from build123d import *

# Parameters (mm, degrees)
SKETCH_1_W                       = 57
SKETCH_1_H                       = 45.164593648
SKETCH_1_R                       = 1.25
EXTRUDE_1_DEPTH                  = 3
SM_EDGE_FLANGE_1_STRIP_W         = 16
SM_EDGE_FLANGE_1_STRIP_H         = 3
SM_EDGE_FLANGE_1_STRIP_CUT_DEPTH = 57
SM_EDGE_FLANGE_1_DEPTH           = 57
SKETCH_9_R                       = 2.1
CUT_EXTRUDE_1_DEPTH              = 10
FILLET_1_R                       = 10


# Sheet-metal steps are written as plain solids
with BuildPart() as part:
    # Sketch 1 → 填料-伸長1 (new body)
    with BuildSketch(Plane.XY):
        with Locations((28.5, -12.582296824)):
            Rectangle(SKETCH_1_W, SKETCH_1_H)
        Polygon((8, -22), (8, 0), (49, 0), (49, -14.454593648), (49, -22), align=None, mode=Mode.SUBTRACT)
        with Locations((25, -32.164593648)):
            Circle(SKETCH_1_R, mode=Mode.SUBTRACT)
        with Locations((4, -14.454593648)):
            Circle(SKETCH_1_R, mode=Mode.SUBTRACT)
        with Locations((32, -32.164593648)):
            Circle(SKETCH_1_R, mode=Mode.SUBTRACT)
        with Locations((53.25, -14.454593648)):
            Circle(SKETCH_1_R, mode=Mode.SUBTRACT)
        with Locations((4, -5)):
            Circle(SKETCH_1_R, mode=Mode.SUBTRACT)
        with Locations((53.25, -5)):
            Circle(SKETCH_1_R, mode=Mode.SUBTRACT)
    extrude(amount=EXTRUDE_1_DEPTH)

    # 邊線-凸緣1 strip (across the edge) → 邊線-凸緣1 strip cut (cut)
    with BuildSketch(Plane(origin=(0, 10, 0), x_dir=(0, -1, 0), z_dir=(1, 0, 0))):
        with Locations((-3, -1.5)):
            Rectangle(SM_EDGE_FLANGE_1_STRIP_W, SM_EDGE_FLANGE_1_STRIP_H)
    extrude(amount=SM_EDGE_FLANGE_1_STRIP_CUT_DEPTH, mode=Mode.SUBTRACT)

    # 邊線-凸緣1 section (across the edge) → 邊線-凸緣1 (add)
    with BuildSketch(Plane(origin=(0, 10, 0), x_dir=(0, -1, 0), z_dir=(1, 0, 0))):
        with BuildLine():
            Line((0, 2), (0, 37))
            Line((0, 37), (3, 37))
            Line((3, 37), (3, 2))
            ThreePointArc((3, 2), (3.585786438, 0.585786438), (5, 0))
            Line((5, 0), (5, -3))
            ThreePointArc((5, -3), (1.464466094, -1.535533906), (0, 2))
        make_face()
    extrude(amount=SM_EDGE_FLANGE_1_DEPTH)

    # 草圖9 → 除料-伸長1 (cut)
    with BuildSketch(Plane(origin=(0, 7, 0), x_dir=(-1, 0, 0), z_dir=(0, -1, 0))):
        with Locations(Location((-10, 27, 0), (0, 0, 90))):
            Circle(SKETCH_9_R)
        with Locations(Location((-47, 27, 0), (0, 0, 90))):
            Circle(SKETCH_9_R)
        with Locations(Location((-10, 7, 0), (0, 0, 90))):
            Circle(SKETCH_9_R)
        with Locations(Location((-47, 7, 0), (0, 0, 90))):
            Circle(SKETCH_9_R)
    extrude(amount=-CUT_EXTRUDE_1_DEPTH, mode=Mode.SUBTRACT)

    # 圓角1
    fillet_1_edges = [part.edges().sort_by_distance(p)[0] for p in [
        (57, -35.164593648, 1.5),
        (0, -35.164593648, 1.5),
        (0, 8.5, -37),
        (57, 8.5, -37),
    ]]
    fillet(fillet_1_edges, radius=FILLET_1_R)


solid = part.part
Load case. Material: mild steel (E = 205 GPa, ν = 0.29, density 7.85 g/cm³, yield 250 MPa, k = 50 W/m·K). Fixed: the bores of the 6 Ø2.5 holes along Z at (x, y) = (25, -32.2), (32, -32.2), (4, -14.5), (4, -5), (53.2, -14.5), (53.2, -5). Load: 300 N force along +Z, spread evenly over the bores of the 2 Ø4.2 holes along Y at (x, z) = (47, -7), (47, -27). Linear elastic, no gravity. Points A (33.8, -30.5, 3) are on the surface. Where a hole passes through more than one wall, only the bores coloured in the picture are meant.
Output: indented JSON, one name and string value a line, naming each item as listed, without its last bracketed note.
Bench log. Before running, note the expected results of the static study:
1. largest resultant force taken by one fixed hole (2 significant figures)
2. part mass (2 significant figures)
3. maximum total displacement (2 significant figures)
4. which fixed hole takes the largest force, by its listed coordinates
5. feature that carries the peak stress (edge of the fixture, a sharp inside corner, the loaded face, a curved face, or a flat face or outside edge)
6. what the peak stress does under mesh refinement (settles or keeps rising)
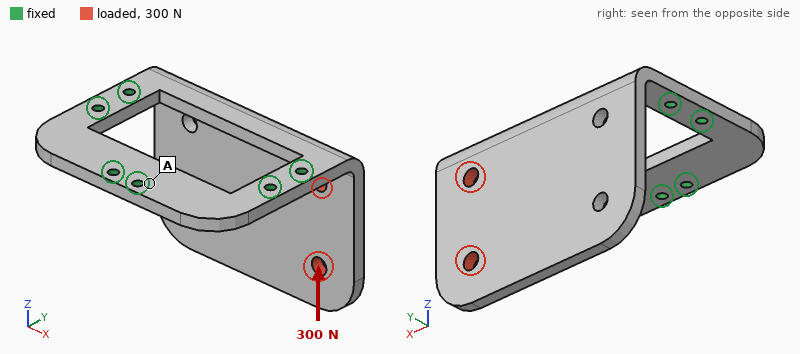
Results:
{
  "largest resultant force taken by one fixed hole": "300 N",
  "part mass": "83 g",
  "maximum total displacement": "0.14 mm",
  "which fixed hole takes the largest force, by its listed coordinates": "(53.2, -5)",
  "feature that carries the peak stress": "edge of the fixture",
  "what the peak stress does under mesh refinement": "keeps rising"
}
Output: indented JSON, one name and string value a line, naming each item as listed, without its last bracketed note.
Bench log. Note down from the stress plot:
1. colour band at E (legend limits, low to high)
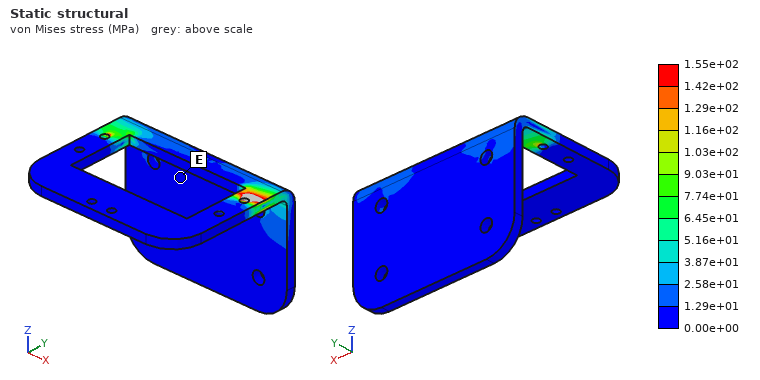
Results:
{
  "colour band at E": "0.00e+00 to 1.29e+01 MPa"
}
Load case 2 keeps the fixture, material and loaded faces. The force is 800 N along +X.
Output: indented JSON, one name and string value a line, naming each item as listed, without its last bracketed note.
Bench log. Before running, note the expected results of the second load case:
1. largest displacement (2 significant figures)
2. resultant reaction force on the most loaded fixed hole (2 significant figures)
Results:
{
  "largest displacement": "63 µm",
  "resultant reaction force on the most loaded fixed hole": "610 N"
}
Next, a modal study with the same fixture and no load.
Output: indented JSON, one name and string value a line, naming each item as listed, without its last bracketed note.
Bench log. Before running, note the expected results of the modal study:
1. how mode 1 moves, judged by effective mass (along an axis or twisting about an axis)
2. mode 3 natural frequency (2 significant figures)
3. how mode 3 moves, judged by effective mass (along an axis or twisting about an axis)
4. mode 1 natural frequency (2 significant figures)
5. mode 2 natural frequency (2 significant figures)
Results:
{
  "how mode 1 moves, judged by effective mass": "along Y",
  "mode 3 natural frequency": "3500 Hz",
  "how mode 3 moves, judged by effective mass": "along Z",
  "mode 1 natural frequency": "750 Hz",
  "mode 2 natural frequency": "2300 Hz"
}
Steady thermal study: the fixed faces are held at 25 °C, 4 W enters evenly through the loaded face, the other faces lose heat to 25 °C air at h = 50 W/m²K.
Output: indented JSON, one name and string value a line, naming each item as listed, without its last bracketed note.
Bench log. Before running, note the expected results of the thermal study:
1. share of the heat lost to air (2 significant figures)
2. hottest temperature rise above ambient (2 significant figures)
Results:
{
  "share of the heat lost to air": "63 %",
  "hottest temperature rise above ambient": "18 K"
}
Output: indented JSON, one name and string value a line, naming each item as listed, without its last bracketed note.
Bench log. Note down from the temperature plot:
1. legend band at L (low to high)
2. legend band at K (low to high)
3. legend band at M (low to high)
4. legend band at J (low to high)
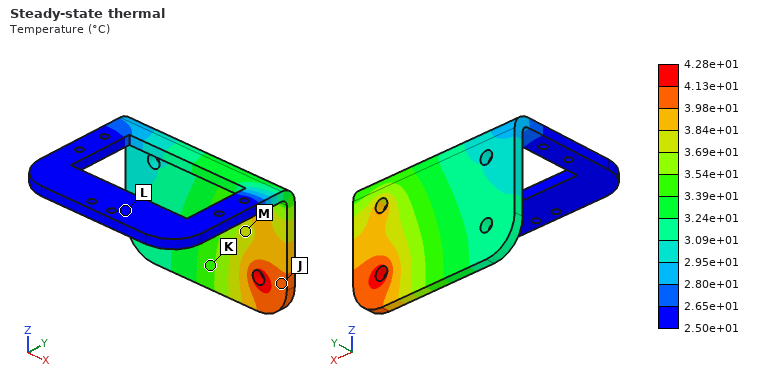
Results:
{
  "legend band at L": "2.50e+01 to 2.65e+01 °C",
  "legend band at K": "3.39e+01 to 3.54e+01 °C",
  "legend band at M": "3.69e+01 to 3.84e+01 °C",
  "legend band at J": "3.98e+01 to 4.13e+01 °C"
}
